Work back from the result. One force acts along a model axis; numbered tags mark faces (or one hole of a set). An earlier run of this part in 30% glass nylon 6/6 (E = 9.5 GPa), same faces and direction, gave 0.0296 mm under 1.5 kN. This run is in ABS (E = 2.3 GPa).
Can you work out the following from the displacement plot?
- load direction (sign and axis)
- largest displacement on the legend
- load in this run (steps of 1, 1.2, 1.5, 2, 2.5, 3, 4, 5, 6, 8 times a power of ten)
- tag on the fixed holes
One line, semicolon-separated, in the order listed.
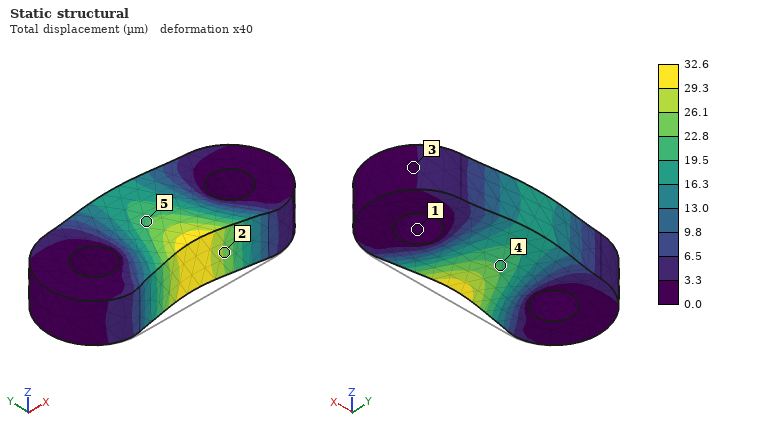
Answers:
+Y; 32.6 µm; 400 N; 1
